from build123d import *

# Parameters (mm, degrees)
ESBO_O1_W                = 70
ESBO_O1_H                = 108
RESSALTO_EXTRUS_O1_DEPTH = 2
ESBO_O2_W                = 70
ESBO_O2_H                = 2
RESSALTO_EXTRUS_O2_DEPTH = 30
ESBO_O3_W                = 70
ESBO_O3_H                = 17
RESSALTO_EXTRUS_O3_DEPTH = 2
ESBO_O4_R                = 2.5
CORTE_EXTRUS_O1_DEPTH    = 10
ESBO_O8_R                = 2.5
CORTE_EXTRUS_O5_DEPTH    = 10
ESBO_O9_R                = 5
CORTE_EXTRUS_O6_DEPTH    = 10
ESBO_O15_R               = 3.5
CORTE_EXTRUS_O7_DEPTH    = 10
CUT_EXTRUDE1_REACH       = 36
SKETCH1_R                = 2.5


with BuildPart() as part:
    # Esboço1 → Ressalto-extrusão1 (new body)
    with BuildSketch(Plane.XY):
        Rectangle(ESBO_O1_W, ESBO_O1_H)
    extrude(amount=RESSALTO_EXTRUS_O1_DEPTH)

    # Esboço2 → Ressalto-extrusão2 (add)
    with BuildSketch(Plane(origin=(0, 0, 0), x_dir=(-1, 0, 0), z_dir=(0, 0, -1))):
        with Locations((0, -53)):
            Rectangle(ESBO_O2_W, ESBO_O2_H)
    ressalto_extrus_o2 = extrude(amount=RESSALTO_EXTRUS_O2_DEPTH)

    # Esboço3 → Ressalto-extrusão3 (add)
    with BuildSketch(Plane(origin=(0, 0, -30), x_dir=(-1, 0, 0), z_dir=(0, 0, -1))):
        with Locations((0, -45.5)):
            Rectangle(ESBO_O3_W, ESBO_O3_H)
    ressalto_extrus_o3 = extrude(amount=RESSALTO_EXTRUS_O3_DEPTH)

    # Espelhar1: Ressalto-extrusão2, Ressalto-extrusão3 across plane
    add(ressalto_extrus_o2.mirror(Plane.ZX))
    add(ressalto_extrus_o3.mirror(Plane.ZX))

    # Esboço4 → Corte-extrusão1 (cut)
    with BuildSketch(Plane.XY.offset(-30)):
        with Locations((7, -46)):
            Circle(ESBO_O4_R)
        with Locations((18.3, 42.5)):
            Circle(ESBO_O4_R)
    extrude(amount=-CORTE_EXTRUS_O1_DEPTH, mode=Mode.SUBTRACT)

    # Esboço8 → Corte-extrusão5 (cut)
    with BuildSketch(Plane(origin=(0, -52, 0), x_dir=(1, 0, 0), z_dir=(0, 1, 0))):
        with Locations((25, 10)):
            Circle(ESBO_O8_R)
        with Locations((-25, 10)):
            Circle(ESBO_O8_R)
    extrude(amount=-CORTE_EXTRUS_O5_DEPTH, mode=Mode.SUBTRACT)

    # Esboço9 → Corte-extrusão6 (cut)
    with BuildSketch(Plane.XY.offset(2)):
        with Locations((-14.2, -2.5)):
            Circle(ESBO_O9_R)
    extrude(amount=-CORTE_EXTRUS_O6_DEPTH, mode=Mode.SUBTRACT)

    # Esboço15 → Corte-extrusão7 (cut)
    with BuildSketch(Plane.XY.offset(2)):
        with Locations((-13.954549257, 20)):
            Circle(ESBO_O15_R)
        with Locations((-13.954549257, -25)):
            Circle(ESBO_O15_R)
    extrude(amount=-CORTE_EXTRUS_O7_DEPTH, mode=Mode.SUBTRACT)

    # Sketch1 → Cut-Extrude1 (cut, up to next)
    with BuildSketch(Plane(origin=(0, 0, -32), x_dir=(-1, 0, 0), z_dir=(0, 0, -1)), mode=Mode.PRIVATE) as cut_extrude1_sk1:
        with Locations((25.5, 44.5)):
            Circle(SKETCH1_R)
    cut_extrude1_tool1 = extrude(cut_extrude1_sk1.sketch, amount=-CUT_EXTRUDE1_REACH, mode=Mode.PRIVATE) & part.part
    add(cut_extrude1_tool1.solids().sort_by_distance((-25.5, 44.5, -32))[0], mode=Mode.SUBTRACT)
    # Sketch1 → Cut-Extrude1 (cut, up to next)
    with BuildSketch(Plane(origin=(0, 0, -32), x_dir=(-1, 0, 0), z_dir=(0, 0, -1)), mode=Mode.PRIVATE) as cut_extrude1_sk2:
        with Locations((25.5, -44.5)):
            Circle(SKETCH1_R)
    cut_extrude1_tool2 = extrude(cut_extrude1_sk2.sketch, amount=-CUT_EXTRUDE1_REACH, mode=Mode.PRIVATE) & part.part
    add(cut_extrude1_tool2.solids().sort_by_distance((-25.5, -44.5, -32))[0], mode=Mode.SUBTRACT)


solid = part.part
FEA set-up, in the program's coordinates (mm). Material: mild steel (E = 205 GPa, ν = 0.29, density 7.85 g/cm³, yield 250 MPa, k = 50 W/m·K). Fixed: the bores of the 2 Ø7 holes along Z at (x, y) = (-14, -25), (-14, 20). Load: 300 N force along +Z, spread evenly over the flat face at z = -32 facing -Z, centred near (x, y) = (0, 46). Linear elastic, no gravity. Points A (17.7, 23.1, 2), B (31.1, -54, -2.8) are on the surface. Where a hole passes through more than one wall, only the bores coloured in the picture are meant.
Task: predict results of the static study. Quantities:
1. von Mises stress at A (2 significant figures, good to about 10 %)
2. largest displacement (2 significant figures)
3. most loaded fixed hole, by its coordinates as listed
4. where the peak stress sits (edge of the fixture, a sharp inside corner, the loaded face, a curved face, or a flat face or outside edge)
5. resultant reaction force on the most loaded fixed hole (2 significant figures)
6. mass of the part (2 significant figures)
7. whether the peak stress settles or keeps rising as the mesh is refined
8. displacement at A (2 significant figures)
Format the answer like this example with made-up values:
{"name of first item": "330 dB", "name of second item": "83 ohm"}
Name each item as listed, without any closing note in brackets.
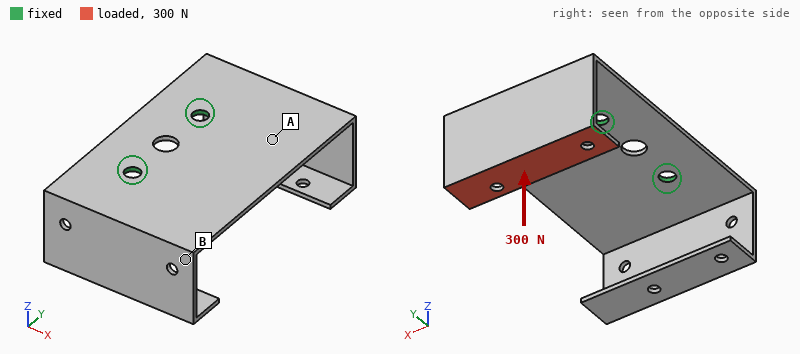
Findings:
{"von Mises stress at A": "70 MPa", "largest displacement": "0.74 mm", "most loaded fixed hole, by its coordinates as listed": "(-14, 20)", "where the peak stress sits": "edge of the fixture", "resultant reaction force on the most loaded fixed hole": "350 N", "mass of the part": "220 g", "whether the peak stress settles or keeps rising as the mesh is refined": "keeps rising", "displacement at A": "0.17 mm"}
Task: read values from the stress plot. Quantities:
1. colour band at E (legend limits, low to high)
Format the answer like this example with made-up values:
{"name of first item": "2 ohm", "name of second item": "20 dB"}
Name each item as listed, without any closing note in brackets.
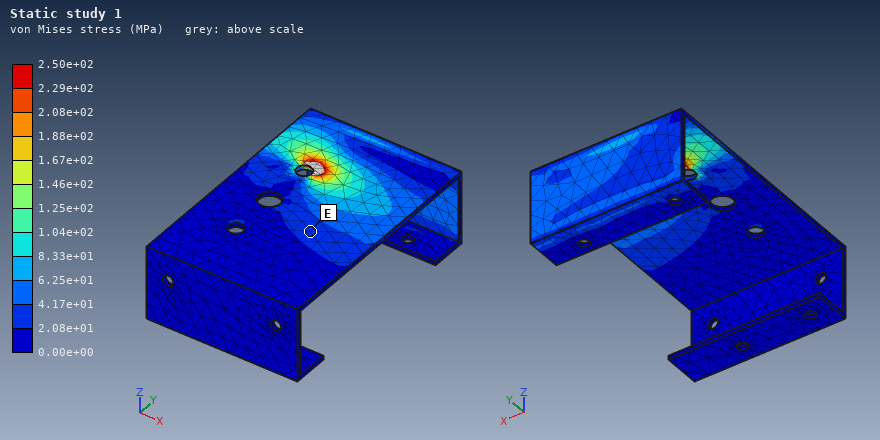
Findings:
{"colour band at E": "2.08e+01 to 4.17e+01 MPa"}
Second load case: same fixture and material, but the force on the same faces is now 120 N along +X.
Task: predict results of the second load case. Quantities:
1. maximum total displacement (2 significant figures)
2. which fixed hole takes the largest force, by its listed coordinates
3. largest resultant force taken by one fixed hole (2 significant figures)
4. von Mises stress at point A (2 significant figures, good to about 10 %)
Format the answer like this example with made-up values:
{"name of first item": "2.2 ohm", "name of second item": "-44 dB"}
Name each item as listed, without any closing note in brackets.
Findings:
{"maximum total displacement": "0.51 mm", "which fixed hole takes the largest force, by its listed coordinates": "(-14, 20)", "largest resultant force taken by one fixed hole": "180 N", "von Mises stress at point A": "33 MPa"}
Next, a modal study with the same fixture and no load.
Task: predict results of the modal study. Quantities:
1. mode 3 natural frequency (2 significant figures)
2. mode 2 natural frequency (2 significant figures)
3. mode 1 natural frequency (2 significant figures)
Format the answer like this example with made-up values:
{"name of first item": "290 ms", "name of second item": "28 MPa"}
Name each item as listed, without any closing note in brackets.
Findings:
{"mode 3 natural frequency": "440 Hz", "mode 2 natural frequency": "380 Hz", "mode 1 natural frequency": "340 Hz"}
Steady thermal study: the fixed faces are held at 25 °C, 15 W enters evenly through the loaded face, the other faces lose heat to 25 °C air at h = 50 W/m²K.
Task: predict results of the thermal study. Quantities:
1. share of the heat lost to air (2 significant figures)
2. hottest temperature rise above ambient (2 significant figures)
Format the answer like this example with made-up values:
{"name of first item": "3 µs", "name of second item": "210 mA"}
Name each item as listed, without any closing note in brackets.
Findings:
{"share of the heat lost to air": "89 %", "hottest temperature rise above ambient": "60 K"}
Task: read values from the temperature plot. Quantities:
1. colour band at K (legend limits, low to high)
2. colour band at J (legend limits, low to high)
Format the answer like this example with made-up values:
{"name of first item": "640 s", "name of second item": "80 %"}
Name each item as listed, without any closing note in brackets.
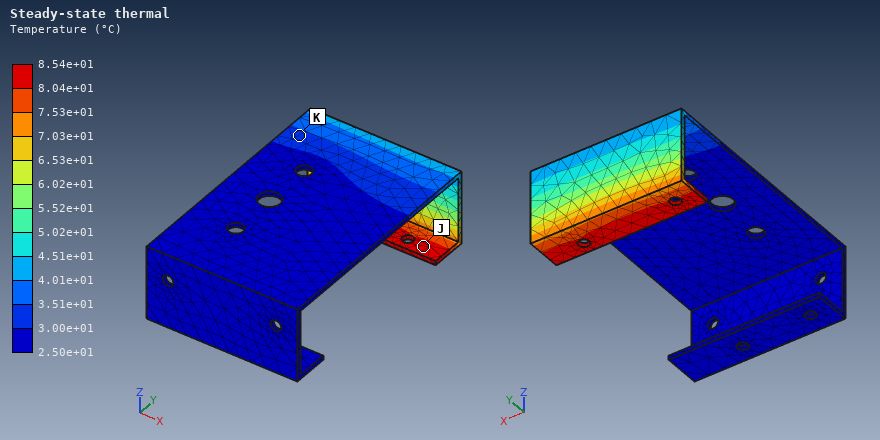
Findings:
{"colour band at K": "3.00e+01 to 3.51e+01 °C", "colour band at J": "8.04e+01 to 8.54e+01 °C"}
